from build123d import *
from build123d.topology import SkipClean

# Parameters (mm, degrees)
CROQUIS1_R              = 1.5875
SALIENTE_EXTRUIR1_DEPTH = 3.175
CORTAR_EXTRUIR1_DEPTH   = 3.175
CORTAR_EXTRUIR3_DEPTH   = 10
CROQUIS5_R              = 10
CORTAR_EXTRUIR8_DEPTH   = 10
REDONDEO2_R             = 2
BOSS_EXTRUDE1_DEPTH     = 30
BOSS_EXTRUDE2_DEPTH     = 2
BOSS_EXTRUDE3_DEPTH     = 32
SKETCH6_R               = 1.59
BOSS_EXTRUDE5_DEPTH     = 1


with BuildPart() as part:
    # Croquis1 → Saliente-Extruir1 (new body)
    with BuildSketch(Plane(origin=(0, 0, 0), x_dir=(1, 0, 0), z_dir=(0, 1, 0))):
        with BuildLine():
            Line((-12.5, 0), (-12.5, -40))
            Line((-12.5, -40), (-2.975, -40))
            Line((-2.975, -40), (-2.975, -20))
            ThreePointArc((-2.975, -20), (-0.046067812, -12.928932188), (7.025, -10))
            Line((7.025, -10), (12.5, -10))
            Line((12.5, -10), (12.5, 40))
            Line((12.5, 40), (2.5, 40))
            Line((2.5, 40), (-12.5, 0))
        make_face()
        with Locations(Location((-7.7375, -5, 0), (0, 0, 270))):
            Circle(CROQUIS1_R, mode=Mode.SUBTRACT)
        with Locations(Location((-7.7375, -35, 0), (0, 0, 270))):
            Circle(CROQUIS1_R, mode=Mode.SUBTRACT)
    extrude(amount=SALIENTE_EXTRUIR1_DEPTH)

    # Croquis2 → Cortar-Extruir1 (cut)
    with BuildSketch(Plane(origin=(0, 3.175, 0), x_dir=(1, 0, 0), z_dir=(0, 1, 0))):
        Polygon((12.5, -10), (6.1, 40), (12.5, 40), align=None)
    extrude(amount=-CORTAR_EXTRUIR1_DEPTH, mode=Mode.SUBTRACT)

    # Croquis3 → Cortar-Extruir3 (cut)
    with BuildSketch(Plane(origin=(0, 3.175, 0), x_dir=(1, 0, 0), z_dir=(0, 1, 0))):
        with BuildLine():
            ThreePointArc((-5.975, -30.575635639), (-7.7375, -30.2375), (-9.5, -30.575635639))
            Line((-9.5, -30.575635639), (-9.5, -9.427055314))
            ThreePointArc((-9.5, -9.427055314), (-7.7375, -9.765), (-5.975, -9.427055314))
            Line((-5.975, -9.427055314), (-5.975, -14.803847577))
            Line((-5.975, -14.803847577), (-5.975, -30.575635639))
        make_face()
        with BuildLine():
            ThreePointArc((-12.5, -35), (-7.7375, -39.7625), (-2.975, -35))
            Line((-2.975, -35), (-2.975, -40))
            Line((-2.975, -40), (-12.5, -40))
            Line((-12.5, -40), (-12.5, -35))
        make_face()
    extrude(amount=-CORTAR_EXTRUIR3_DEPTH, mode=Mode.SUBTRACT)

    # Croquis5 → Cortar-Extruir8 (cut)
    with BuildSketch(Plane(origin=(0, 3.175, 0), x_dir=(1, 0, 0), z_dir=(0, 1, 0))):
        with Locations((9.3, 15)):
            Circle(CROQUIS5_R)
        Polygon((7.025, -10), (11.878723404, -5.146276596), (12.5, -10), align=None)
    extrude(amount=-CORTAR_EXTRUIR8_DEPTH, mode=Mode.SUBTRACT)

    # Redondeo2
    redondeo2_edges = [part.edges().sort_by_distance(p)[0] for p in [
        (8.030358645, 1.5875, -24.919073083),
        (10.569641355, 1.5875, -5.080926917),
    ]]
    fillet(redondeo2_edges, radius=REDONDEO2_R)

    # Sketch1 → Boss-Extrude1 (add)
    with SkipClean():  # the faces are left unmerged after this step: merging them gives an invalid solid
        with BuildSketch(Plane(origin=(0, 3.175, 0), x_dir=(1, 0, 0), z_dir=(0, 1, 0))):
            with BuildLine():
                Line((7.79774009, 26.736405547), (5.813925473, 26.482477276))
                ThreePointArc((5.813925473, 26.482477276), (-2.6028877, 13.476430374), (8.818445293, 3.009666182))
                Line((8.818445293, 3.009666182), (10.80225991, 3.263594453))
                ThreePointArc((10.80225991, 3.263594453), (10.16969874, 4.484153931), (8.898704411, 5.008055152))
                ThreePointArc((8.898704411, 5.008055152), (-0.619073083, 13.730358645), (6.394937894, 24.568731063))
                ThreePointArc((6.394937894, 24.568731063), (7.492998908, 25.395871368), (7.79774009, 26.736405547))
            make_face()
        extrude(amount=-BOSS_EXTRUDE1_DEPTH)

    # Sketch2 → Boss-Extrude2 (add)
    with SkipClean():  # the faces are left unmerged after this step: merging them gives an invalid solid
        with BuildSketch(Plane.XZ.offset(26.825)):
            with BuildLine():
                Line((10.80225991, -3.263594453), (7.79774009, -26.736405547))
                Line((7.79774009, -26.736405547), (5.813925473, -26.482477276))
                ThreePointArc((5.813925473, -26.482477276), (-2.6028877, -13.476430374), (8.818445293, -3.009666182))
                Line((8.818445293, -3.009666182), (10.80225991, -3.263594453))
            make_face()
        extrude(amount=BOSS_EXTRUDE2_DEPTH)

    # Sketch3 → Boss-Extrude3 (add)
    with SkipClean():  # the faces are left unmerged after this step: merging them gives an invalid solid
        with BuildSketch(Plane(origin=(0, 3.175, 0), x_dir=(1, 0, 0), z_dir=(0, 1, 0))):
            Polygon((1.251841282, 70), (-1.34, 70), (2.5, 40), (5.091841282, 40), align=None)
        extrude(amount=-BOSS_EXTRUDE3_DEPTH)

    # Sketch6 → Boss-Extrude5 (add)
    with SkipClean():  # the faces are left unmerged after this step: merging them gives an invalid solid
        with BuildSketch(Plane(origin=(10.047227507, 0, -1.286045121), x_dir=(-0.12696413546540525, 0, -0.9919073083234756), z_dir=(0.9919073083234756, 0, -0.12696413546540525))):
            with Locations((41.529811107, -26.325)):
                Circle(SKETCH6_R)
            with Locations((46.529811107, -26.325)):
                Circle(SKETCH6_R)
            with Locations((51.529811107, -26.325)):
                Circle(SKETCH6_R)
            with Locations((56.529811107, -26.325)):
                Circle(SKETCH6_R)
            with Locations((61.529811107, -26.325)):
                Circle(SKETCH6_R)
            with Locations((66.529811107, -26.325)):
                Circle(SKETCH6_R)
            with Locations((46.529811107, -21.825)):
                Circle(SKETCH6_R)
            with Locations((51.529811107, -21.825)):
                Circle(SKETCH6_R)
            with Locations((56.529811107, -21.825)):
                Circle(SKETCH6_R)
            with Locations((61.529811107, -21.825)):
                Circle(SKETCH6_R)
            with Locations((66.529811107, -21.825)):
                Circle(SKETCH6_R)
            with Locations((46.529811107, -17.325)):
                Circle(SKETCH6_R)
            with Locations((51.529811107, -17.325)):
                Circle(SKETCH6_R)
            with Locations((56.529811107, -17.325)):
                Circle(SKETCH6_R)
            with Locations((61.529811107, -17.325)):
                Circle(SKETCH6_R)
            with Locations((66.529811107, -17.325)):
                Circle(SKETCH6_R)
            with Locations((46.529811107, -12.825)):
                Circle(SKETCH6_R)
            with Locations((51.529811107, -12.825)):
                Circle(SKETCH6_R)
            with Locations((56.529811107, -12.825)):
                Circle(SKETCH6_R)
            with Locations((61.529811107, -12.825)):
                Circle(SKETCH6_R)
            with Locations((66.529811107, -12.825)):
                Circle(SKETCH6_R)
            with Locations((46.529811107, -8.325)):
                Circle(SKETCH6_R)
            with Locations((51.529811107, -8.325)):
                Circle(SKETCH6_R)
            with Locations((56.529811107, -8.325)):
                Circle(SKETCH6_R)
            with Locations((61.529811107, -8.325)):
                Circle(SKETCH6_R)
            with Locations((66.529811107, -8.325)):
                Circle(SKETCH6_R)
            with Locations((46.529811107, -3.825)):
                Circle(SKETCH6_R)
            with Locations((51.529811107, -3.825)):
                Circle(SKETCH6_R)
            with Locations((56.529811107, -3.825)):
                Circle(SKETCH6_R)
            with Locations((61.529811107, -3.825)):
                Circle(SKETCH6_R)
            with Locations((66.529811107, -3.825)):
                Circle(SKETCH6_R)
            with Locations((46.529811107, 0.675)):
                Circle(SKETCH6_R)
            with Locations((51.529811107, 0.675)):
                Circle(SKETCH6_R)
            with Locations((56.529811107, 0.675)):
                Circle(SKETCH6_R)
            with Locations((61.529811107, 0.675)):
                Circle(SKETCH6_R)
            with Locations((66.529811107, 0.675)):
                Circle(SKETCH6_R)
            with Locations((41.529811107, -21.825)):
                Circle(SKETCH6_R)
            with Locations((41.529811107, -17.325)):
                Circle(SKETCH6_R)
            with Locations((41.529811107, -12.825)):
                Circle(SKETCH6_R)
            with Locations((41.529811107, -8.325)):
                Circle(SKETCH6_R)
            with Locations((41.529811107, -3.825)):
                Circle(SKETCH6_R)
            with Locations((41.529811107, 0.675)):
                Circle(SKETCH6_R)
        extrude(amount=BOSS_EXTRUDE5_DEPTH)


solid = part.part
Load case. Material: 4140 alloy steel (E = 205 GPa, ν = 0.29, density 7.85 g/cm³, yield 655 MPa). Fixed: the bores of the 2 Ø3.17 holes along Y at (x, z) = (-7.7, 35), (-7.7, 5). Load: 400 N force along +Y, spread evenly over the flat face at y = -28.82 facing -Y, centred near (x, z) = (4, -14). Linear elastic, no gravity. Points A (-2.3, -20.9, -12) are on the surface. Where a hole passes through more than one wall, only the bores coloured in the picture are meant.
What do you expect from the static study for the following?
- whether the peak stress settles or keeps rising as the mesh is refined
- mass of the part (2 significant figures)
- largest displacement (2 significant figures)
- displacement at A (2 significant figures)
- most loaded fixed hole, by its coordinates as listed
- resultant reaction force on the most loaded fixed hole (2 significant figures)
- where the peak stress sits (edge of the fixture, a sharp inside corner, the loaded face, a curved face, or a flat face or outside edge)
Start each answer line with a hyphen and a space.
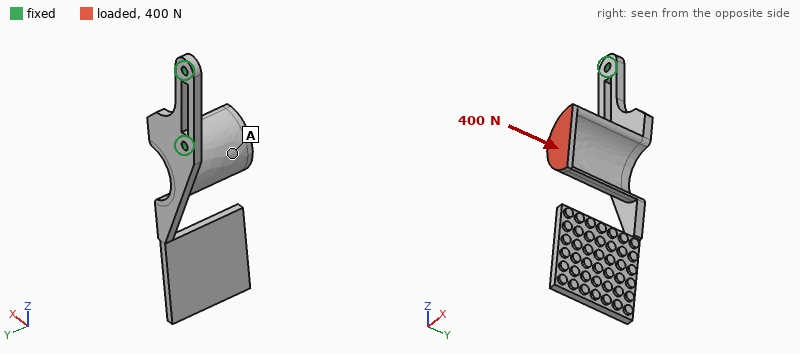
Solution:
- keeps rising
- 60 g
- 0.75 mm
- 0.27 mm
- (-7.7, 5)
- 450 N
- edge of the fixture
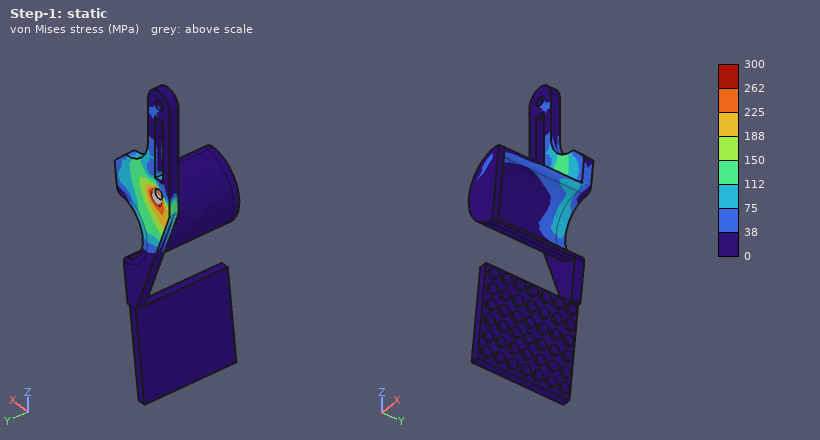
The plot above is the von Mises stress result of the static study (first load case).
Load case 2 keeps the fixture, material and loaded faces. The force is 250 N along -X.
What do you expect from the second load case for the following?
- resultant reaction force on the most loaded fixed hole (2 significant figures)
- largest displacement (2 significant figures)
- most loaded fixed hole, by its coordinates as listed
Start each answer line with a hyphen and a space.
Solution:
- 300 N
- 0.54 mm
- (-7.7, 5)
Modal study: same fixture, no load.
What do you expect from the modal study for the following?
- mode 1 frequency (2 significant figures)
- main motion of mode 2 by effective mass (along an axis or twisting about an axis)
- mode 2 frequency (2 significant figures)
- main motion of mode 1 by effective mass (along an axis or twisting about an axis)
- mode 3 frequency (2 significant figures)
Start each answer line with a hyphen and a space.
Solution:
- 310 Hz
- along X
- 440 Hz
- along Y
- 1000 Hz
